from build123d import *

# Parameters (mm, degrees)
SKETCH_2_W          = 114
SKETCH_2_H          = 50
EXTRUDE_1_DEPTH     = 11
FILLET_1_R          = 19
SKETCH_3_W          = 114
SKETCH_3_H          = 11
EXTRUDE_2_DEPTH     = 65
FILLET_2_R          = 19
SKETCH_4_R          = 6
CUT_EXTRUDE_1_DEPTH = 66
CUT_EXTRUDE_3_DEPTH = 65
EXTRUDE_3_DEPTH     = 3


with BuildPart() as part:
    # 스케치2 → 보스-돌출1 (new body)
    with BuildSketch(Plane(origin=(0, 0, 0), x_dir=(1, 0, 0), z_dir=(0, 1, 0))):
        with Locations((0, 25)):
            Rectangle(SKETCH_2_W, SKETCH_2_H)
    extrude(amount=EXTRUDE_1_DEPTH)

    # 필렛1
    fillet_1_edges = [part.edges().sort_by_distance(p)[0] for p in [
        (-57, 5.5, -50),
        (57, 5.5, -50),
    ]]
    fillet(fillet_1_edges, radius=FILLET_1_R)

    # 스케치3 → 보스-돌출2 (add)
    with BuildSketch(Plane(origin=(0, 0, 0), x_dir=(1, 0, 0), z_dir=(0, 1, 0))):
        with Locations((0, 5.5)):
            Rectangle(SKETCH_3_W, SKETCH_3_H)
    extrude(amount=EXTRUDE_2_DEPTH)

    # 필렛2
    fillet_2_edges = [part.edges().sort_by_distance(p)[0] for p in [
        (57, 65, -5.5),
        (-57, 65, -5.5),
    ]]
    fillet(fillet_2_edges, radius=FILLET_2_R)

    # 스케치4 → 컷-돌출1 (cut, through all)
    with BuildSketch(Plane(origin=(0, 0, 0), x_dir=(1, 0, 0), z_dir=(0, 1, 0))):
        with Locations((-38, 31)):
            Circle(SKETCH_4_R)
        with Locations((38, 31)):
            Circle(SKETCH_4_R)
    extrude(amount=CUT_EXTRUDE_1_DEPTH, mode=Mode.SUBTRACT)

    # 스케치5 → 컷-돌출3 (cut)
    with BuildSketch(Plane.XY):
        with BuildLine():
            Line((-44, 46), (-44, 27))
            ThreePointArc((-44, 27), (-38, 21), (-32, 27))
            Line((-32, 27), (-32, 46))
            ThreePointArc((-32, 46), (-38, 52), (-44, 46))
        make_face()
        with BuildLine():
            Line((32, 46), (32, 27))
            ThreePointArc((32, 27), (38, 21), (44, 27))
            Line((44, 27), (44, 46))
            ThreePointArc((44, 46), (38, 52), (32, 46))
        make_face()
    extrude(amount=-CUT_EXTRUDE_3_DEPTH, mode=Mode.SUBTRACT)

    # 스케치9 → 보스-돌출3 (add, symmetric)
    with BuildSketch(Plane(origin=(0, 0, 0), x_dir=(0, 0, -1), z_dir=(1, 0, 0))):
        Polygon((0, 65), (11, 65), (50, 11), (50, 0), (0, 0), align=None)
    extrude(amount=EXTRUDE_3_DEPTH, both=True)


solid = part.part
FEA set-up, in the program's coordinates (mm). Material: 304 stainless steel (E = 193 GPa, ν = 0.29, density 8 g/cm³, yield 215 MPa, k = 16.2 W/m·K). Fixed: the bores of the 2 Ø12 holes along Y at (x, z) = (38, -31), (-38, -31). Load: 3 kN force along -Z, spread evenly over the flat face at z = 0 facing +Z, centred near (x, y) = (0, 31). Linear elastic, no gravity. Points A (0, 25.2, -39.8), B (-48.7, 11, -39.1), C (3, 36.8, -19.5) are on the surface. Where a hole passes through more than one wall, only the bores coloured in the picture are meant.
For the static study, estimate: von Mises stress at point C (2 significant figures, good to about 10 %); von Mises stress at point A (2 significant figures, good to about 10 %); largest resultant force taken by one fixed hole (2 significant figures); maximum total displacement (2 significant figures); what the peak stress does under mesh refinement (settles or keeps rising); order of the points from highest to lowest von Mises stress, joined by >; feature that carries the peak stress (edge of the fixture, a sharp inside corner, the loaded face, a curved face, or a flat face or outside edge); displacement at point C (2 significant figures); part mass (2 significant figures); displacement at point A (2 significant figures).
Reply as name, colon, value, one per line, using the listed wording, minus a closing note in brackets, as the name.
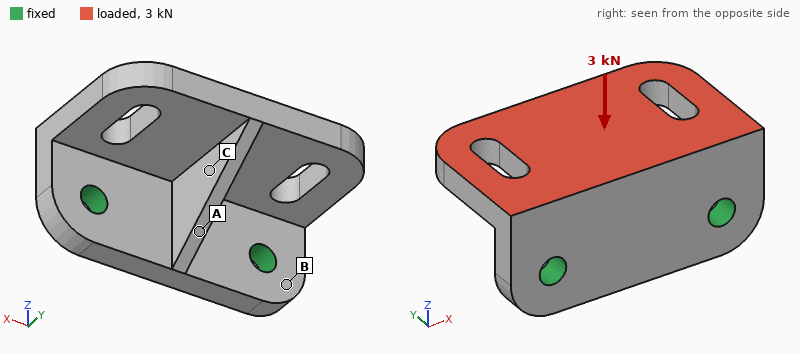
von Mises stress at point C: 12 MPa
von Mises stress at point A: 19 MPa
largest resultant force taken by one fixed hole: 1.5 kN
maximum total displacement: 42 µm
what the peak stress does under mesh refinement: keeps rising
order of the points from highest to lowest von Mises stress, joined by >: A > C > B
feature that carries the peak stress: edge of the fixture
displacement at point C: 18 µm
part mass: 990 g
displacement at point A: 13 µm
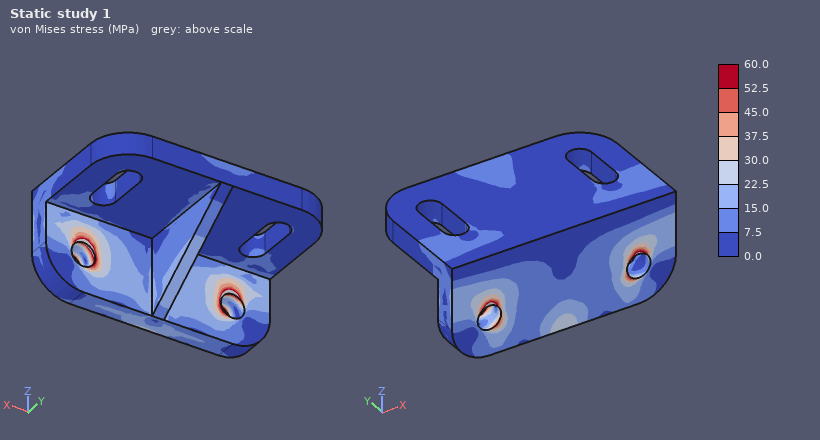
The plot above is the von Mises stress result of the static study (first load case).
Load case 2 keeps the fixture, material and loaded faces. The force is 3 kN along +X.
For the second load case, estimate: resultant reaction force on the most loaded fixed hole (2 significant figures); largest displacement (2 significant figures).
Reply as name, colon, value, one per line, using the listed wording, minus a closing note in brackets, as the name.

resultant reaction force on the most loaded fixed hole: 2.1 kN
largest displacement: 7.1 µm
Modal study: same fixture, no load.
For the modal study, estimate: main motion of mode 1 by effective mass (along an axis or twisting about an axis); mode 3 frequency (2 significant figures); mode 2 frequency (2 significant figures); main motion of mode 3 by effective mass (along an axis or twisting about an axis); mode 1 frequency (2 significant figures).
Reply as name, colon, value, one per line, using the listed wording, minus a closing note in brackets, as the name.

main motion of mode 1 by effective mass: along Z
mode 3 frequency: 4800 Hz
mode 2 frequency: 3100 Hz
main motion of mode 3 by effective mass: along X
mode 1 frequency: 2000 Hz
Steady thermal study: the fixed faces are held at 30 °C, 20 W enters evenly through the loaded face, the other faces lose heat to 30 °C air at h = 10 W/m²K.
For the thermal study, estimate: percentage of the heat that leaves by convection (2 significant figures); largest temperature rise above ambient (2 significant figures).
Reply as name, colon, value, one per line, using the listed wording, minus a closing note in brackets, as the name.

percentage of the heat that leaves by convection: 24 %
largest temperature rise above ambient: 40 K
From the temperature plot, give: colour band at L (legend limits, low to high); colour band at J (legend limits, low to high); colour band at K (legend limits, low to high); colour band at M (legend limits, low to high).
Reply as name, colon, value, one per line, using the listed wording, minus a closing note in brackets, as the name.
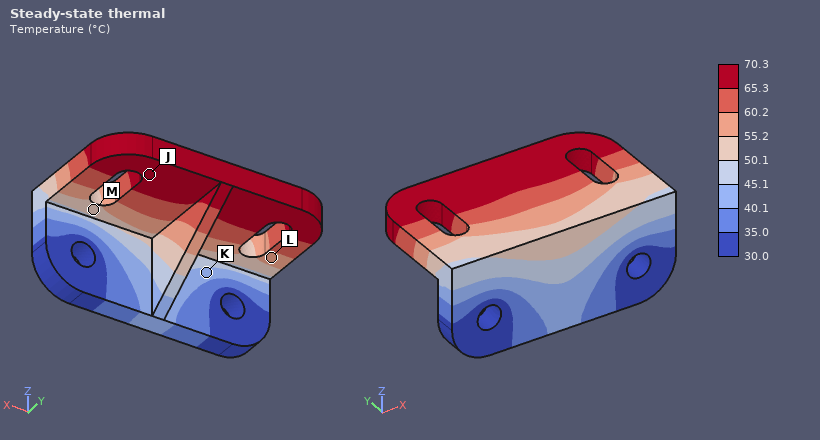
colour band at L: 55.2 to 60.2 °C
colour band at J: 65.3 to 70.3 °C
colour band at K: 40.1 to 45.1 °C
colour band at M: 50.1 to 55.2 °C
